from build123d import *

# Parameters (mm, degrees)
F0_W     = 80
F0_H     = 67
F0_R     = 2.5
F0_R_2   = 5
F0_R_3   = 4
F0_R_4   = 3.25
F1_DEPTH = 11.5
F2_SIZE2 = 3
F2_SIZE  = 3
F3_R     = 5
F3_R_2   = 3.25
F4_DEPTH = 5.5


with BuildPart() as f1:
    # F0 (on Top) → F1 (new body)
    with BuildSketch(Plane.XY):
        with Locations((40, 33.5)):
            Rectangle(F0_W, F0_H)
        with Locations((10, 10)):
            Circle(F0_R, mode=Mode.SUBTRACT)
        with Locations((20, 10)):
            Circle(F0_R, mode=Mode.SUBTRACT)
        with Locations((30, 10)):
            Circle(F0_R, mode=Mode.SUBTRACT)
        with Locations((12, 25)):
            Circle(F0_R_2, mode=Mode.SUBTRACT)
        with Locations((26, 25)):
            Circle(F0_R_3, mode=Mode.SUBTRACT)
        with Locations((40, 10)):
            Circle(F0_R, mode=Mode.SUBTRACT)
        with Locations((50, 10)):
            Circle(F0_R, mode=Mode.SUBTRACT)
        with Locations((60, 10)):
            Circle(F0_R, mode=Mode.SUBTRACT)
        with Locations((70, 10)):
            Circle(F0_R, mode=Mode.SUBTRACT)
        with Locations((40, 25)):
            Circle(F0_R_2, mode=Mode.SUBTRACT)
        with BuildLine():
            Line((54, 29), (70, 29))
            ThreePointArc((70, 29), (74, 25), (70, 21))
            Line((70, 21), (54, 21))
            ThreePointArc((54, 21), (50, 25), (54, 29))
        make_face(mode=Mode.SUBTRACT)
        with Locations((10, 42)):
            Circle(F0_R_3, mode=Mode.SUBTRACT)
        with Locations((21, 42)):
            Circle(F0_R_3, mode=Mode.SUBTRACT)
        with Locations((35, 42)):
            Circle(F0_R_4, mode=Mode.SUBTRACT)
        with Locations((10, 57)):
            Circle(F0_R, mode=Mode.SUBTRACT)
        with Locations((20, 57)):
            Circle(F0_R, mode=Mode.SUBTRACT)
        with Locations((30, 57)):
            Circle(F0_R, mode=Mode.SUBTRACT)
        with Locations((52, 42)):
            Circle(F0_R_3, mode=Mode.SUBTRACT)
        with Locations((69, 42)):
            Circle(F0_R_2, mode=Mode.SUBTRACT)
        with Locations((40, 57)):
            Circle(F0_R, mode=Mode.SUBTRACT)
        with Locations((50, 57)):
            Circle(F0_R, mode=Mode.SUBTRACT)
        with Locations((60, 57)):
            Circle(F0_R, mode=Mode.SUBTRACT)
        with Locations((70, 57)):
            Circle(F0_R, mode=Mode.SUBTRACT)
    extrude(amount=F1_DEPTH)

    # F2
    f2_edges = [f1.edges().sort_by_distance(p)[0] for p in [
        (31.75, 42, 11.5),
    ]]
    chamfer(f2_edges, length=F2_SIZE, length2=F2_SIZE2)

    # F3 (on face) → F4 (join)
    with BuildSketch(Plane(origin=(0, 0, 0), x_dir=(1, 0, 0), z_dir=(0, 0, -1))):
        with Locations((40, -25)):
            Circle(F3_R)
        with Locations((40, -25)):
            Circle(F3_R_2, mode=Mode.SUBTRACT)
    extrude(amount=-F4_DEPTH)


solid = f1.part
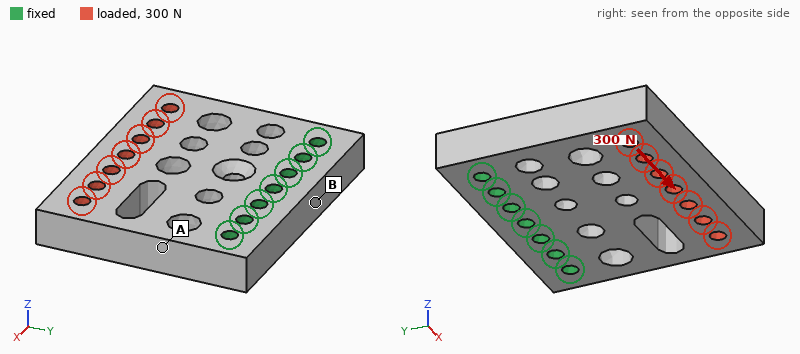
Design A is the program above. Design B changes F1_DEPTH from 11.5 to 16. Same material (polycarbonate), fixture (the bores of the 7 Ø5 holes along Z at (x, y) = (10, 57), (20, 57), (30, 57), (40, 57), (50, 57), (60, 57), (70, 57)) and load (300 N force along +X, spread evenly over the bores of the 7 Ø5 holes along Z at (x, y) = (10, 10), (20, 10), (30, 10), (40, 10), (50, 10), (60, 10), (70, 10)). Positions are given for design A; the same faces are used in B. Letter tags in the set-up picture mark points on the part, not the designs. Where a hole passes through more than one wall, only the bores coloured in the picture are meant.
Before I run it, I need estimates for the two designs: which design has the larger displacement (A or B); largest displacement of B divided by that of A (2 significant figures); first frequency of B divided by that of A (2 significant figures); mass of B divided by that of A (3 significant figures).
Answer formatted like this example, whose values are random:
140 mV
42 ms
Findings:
A
0.72
1.3
1.39
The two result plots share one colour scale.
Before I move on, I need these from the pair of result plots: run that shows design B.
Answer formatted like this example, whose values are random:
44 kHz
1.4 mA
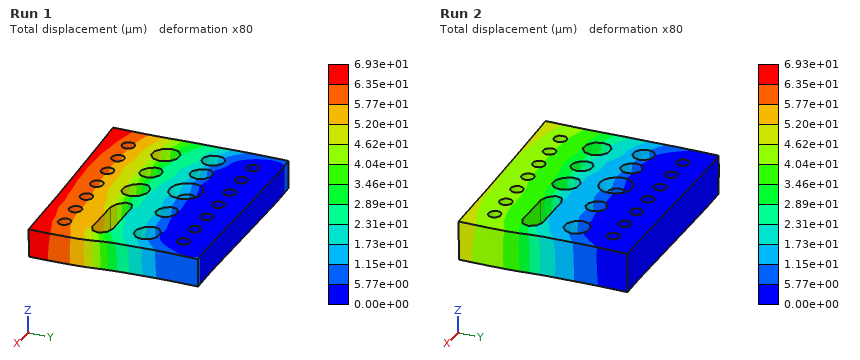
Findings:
Run 2
